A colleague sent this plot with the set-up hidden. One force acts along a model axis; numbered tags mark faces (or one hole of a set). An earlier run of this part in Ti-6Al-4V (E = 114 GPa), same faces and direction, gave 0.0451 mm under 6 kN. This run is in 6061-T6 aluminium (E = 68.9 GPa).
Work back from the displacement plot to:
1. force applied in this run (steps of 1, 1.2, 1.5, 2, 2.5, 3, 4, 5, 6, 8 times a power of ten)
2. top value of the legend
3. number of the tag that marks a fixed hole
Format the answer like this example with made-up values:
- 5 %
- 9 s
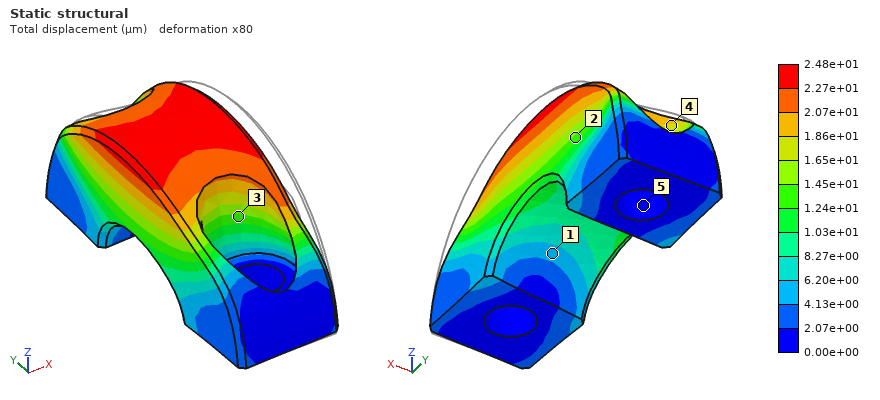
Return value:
- 2 kN
- 2.48e+01 µm
- 5
